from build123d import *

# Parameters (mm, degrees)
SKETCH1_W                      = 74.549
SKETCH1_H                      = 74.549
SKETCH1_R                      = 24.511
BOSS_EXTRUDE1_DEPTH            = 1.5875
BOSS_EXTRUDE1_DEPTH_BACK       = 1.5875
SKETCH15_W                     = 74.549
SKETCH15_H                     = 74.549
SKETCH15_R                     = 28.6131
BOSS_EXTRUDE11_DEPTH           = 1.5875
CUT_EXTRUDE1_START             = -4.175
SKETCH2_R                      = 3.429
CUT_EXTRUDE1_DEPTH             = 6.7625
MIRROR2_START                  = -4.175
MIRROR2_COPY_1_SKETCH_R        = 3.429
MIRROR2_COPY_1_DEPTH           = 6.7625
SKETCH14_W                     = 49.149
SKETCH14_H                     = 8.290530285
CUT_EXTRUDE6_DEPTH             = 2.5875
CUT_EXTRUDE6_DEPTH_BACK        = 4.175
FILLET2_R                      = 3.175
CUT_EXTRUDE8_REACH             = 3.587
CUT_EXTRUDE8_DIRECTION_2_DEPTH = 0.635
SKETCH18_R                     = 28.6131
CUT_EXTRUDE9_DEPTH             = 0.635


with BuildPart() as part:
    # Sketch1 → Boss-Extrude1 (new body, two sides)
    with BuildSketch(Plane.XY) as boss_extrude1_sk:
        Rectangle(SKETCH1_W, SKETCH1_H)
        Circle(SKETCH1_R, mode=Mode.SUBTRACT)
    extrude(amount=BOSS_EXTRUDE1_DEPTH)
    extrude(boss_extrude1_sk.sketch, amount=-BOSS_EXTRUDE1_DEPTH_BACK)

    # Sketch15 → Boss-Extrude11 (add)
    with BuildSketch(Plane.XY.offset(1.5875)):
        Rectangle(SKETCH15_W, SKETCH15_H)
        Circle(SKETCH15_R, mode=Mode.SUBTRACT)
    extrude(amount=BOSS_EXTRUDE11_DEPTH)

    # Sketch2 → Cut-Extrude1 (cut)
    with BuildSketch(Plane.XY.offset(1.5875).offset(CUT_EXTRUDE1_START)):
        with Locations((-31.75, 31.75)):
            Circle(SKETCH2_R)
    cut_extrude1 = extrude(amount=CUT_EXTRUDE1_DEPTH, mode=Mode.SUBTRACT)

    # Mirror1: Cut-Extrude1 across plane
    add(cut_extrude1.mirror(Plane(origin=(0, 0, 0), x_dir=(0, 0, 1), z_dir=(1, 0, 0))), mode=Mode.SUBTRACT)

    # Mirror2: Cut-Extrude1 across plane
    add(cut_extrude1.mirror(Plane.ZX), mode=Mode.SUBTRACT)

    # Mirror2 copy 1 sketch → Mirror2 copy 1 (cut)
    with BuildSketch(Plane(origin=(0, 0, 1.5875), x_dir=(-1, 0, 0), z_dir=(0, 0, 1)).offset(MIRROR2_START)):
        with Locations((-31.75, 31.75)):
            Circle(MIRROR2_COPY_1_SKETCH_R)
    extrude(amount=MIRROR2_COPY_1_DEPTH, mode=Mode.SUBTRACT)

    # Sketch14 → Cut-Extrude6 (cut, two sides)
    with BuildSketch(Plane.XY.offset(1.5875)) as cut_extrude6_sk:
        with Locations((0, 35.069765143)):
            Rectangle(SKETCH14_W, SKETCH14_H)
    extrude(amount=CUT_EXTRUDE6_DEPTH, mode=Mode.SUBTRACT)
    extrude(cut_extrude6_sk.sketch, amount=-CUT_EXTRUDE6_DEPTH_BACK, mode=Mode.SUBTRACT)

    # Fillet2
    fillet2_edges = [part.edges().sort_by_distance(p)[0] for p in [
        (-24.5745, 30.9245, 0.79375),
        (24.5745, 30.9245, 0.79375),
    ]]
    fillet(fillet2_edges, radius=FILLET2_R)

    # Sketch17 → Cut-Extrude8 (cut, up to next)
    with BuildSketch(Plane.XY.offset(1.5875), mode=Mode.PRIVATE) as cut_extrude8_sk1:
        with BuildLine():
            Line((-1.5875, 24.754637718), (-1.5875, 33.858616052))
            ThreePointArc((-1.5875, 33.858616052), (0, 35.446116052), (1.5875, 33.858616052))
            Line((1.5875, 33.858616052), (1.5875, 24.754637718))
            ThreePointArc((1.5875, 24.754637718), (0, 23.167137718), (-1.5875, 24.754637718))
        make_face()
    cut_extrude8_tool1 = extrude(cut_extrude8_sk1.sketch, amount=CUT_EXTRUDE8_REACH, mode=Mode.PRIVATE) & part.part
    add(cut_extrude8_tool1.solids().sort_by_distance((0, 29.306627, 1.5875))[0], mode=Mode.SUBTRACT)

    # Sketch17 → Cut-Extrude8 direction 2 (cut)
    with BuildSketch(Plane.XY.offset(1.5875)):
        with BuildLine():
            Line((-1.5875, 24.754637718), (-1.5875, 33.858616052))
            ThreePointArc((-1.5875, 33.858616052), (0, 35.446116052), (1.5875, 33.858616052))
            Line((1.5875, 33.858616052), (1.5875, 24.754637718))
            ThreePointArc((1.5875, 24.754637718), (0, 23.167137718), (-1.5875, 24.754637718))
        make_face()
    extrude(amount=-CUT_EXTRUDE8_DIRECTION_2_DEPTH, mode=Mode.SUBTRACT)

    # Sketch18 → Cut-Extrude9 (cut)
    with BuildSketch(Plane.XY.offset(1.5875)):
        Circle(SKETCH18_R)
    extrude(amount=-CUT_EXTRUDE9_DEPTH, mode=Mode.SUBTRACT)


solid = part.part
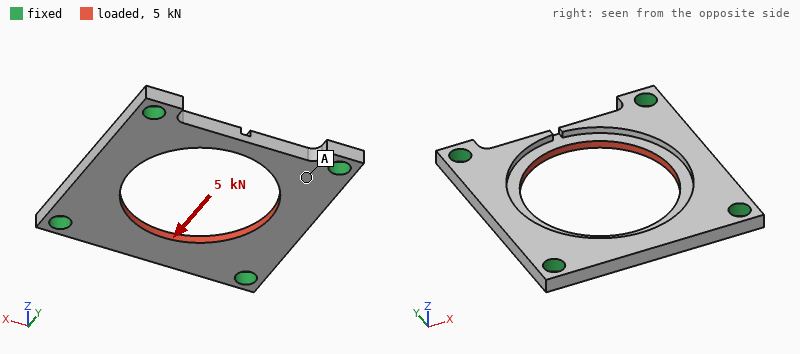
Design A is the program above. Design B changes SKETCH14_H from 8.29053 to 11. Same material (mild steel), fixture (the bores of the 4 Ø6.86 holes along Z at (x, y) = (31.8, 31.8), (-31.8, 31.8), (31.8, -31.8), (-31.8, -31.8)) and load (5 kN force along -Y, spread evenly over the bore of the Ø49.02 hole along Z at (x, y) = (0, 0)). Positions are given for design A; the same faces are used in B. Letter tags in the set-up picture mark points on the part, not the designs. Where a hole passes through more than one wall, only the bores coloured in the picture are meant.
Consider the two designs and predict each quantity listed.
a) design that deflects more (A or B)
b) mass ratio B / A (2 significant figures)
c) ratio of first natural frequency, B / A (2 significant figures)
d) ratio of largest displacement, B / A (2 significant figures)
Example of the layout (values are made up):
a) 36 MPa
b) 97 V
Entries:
a) B
b) 0.98
c) 1.00
d) 1.3
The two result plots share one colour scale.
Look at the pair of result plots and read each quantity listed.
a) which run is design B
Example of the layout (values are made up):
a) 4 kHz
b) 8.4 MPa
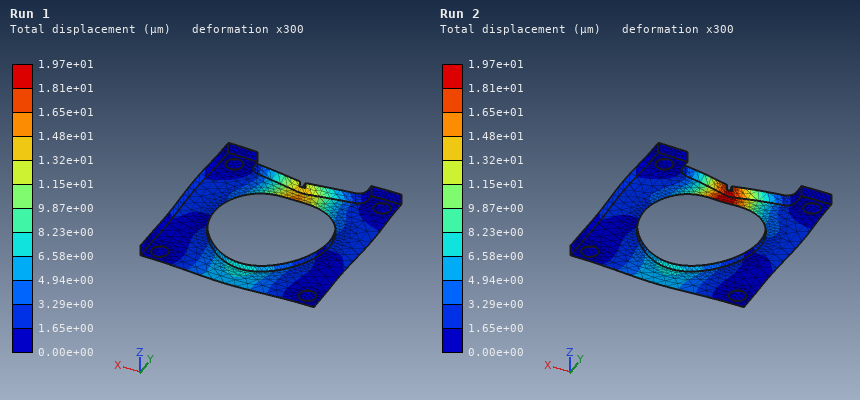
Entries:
a) Run 2
